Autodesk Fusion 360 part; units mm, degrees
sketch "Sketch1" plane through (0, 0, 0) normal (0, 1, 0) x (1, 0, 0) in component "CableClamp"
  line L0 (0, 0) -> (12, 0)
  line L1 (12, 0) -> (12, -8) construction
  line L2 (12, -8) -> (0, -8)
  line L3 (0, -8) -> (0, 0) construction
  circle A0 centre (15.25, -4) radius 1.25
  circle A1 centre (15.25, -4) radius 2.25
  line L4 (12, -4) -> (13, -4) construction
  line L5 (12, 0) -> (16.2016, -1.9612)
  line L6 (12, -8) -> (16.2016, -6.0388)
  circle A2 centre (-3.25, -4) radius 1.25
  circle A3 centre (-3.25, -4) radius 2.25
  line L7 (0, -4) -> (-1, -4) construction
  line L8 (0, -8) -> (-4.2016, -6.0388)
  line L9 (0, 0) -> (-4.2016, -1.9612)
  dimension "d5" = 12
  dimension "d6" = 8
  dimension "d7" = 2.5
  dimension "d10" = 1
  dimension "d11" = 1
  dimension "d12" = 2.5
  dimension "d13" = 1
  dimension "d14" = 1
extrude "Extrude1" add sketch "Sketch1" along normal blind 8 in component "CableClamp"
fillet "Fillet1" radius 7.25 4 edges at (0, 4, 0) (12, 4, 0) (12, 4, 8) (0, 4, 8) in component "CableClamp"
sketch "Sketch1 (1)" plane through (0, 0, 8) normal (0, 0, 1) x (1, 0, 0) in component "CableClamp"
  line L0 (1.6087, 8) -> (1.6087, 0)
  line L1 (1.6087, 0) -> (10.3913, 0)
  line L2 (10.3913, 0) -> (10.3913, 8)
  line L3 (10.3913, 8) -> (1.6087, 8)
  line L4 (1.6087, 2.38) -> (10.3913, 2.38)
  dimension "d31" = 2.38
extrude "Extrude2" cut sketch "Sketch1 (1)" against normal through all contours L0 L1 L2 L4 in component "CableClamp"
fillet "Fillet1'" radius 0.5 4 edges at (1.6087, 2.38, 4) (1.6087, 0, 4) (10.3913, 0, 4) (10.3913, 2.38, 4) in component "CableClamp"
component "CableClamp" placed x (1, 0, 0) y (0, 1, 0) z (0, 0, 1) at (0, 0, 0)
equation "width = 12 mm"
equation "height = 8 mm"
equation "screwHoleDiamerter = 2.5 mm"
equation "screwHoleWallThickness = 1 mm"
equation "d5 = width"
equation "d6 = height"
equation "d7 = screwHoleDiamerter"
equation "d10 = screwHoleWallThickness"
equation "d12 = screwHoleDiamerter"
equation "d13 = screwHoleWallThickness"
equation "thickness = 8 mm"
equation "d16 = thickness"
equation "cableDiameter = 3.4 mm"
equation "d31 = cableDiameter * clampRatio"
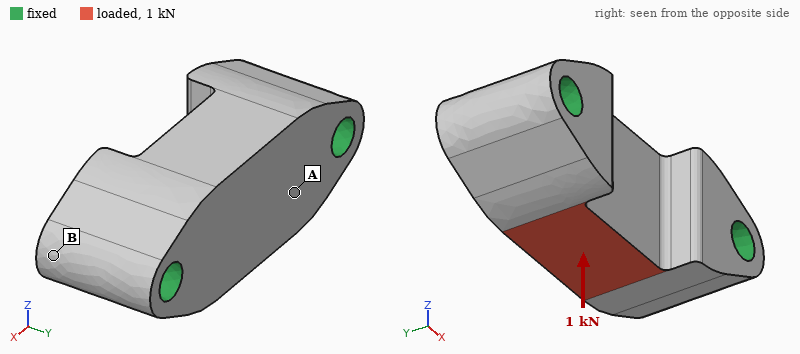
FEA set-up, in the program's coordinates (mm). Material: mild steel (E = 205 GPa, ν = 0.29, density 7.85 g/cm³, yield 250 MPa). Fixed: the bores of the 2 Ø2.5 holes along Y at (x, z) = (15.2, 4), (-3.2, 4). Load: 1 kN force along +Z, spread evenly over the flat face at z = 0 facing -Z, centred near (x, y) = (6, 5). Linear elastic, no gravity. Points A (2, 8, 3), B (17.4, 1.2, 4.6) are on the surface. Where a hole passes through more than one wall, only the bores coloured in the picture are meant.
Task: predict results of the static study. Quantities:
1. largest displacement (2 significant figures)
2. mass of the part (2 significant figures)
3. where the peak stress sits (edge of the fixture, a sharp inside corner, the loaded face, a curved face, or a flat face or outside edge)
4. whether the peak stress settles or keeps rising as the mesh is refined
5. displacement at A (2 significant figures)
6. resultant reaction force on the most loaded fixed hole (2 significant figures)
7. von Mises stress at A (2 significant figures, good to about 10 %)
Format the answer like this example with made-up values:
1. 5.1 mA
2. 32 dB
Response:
1. 2.4 µm
2. 7.7 g
3. edge of the fixture
4. keeps rising
5. 1.5 µm
6. 500 N
7. 28 MPa
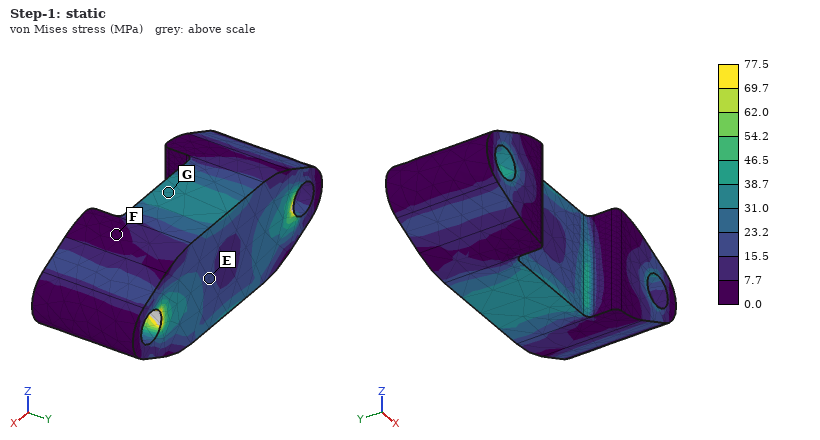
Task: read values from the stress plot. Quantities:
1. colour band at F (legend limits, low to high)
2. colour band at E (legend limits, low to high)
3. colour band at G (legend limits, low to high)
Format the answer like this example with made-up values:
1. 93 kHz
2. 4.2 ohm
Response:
1. 0.0 to 7.7 MPa
2. 15.5 to 23.2 MPa
3. 31.0 to 38.7 MPa
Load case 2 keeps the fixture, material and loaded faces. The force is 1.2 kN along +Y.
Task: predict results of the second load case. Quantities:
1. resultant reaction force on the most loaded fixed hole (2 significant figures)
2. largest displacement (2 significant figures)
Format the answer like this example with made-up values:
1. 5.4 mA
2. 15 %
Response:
1. 620 N
2. 5.5 µm
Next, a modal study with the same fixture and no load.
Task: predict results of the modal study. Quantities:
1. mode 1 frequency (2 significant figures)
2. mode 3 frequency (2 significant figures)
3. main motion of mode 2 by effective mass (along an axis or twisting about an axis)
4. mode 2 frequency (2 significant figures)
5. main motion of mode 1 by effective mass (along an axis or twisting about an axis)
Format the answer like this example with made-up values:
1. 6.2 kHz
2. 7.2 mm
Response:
1. 60 kHz
2. 88 kHz
3. along Y
4. 71 kHz
5. along Z
